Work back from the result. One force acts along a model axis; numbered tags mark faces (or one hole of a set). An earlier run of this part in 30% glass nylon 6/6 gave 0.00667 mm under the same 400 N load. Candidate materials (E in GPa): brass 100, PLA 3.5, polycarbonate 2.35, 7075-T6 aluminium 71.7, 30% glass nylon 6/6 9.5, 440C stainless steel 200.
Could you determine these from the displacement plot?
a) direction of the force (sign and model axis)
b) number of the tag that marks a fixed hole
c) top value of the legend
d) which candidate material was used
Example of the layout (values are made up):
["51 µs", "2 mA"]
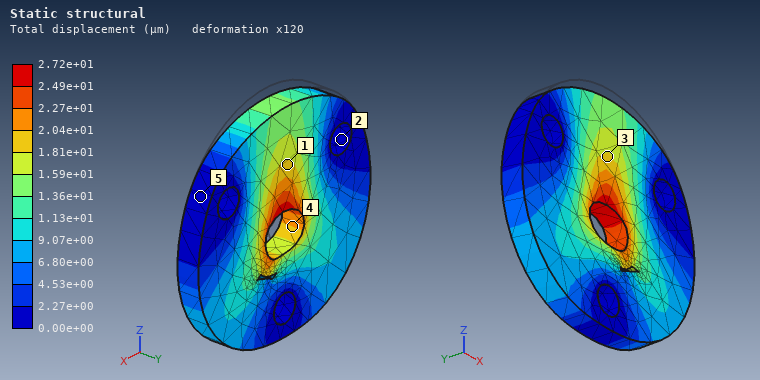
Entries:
["-Z", "2", "2.72e+01 µm", "polycarbonate"]
